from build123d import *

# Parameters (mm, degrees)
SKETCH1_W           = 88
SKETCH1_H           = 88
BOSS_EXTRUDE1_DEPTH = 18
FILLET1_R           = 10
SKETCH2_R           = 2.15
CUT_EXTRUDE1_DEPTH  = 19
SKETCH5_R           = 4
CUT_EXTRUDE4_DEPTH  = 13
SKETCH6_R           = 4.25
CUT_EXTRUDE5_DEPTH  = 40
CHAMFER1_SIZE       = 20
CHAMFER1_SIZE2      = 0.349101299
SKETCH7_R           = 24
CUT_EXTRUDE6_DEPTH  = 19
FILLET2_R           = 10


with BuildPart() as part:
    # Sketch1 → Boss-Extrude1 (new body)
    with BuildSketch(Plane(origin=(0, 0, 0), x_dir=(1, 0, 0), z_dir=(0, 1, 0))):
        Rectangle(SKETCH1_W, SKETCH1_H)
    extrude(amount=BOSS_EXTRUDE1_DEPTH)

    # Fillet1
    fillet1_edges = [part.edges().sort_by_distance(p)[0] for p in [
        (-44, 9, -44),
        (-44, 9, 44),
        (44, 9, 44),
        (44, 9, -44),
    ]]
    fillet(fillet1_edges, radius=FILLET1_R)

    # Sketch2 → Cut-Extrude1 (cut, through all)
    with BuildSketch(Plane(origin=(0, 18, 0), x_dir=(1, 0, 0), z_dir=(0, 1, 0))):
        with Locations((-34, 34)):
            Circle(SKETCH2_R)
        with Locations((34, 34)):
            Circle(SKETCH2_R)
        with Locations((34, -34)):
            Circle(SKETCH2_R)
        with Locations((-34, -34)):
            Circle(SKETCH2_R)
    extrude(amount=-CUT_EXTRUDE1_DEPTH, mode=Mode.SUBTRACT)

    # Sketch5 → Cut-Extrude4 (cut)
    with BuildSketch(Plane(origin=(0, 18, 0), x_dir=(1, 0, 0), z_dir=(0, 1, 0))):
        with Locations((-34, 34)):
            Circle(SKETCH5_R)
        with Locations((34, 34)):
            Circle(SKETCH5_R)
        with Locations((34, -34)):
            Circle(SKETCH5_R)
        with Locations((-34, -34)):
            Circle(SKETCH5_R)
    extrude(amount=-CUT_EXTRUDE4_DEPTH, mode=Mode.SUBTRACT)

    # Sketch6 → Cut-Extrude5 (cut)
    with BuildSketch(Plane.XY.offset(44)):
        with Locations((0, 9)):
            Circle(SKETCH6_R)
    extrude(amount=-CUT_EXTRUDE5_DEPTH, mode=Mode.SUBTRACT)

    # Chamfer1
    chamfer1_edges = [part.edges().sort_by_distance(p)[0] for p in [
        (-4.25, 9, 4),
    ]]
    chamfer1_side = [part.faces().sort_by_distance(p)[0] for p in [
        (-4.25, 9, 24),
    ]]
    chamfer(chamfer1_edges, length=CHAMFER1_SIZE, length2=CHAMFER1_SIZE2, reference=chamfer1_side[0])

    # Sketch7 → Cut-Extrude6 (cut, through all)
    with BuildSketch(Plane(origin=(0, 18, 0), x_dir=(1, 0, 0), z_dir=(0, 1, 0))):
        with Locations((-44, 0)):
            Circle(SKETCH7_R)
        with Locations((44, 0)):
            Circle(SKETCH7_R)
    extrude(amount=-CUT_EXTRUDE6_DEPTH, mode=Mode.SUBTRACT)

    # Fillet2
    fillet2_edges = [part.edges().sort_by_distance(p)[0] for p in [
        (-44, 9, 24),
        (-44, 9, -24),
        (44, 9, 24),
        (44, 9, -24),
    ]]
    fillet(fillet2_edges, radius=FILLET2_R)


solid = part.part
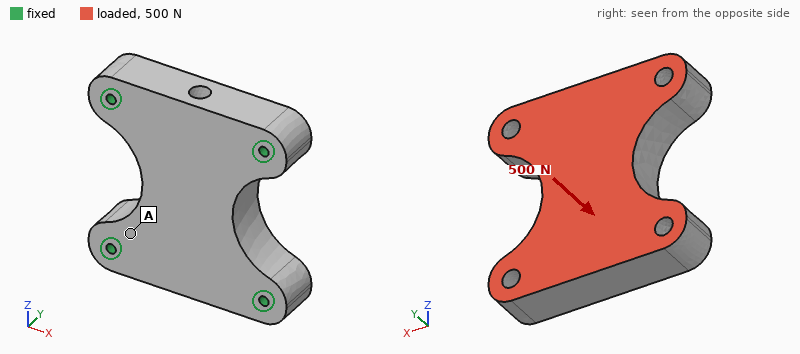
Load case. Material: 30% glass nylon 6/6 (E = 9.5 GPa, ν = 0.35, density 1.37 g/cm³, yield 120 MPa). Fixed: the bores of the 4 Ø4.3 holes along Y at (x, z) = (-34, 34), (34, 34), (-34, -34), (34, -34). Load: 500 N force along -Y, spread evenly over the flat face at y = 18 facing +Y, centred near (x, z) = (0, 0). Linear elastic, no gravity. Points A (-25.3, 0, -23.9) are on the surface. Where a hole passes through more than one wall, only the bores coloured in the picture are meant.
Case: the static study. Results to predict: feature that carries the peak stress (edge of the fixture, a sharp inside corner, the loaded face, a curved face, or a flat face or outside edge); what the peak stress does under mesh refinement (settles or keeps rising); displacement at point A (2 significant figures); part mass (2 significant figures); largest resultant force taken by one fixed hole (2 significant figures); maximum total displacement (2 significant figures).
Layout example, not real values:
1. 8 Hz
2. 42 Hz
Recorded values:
1. edge of the fixture
2. keeps rising
3. 4.7 µm
4. 140 g
5. 150 N
6. 8.4 µm
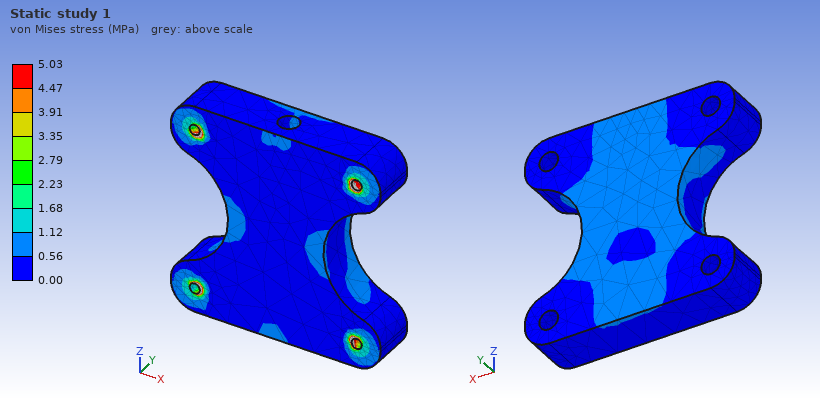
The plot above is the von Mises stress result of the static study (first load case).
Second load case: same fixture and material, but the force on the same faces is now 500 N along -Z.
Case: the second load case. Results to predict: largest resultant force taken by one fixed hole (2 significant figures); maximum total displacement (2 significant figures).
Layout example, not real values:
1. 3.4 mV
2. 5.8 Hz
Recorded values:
1. 150 N
2. 7.9 µm
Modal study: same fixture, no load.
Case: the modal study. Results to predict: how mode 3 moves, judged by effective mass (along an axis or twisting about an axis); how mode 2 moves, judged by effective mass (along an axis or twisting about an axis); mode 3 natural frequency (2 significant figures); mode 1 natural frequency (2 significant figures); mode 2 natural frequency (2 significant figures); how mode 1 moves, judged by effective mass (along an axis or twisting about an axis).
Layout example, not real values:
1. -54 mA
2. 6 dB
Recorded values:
1. along Z
2. along Z
3. 5500 Hz
4. 3800 Hz
5. 5000 Hz
6. along Y
